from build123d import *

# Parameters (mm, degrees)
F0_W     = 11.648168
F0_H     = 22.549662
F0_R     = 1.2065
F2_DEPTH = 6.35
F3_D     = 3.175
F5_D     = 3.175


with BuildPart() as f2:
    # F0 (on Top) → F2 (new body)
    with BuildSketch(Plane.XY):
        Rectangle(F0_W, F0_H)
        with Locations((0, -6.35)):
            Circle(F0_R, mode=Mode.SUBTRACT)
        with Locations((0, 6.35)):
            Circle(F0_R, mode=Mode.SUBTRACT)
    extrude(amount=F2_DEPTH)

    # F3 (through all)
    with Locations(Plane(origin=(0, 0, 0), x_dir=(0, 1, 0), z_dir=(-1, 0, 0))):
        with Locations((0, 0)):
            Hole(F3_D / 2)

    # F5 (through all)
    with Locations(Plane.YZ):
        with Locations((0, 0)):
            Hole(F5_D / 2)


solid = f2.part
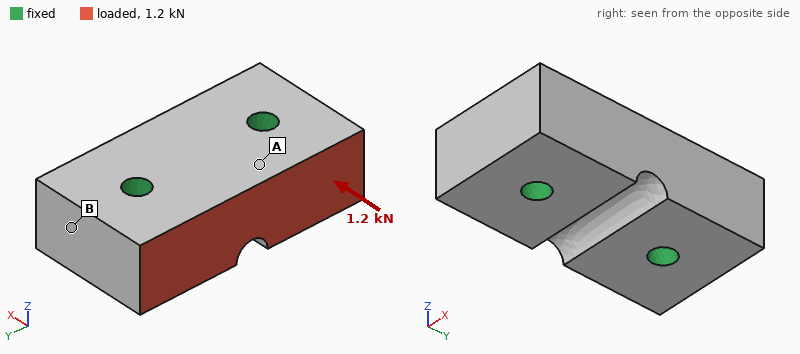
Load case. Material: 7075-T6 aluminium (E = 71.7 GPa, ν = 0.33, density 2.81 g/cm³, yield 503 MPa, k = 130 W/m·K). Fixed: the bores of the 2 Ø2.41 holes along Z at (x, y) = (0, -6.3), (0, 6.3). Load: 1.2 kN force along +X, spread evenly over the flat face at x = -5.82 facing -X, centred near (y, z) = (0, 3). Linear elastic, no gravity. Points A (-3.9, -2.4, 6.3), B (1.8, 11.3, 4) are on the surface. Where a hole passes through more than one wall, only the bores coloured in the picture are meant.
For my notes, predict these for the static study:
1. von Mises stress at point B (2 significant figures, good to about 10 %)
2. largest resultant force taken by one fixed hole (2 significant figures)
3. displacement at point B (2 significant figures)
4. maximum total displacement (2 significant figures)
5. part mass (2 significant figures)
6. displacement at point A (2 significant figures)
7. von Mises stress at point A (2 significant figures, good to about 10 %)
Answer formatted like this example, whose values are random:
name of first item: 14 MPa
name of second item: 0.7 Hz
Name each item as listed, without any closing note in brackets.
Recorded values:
von Mises stress at point B: 3.8 MPa
largest resultant force taken by one fixed hole: 600 N
displacement at point B: 0.48 µm
maximum total displacement: 1.3 µm
part mass: 4.4 g
displacement at point A: 0.85 µm
von Mises stress at point A: 8.1 MPa
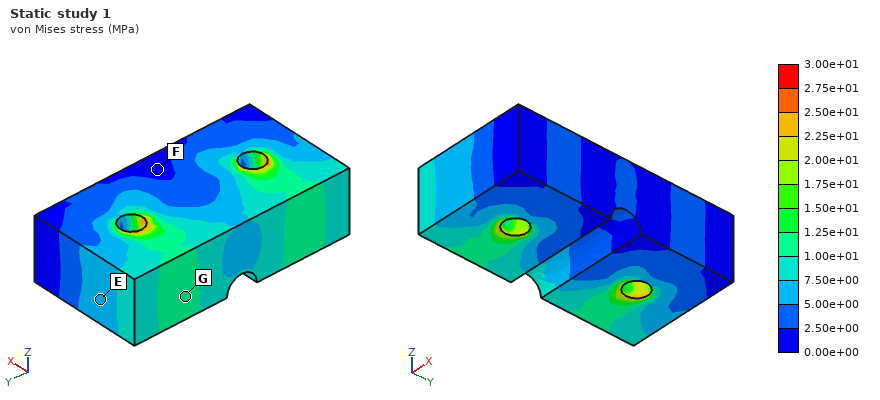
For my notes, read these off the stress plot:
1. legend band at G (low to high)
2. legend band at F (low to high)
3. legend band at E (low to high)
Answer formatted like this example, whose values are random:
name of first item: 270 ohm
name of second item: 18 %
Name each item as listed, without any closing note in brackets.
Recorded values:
legend band at G: 1.00e+01 to 1.25e+01 MPa
legend band at F: 0.00e+00 to 2.50e+00 MPa
legend band at E: 5.00e+00 to 7.50e+00 MPa
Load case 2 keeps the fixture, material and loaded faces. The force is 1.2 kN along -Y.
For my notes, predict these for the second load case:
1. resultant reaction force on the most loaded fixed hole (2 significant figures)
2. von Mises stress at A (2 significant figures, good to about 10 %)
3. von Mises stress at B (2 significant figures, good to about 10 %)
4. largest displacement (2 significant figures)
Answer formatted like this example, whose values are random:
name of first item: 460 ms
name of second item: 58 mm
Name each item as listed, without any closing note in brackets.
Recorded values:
resultant reaction force on the most loaded fixed hole: 740 N
von Mises stress at A: 21 MPa
von Mises stress at B: 8.9 MPa
largest displacement: 4.8 µm
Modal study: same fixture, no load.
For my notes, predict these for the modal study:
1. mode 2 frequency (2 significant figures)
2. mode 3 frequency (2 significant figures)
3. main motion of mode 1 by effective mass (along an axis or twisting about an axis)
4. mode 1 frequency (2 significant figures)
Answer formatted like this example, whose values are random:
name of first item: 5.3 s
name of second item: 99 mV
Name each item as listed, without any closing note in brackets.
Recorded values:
mode 2 frequency: 82 kHz
mode 3 frequency: 84 kHz
main motion of mode 1 by effective mass: twisting about Y
mode 1 frequency: 74 kHz
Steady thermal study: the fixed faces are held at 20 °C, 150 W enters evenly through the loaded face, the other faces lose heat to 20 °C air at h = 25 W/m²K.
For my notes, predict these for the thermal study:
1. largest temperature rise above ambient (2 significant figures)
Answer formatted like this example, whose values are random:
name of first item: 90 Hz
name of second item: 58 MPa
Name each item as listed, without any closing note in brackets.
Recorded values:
largest temperature rise above ambient: 56 K
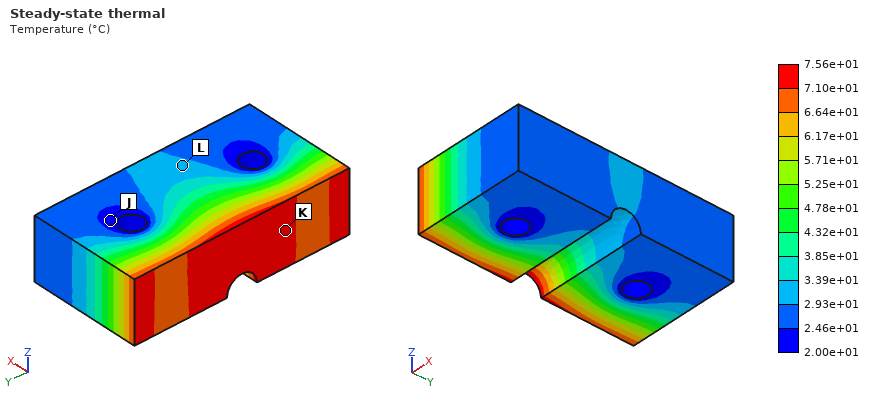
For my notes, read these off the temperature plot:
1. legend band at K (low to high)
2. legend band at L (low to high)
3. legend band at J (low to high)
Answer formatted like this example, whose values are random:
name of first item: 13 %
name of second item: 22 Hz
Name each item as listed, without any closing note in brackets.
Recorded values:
legend band at K: 7.10e+01 to 7.56e+01 °C
legend band at L: 2.93e+01 to 3.39e+01 °C
legend band at J: 2.00e+01 to 2.46e+01 °C
